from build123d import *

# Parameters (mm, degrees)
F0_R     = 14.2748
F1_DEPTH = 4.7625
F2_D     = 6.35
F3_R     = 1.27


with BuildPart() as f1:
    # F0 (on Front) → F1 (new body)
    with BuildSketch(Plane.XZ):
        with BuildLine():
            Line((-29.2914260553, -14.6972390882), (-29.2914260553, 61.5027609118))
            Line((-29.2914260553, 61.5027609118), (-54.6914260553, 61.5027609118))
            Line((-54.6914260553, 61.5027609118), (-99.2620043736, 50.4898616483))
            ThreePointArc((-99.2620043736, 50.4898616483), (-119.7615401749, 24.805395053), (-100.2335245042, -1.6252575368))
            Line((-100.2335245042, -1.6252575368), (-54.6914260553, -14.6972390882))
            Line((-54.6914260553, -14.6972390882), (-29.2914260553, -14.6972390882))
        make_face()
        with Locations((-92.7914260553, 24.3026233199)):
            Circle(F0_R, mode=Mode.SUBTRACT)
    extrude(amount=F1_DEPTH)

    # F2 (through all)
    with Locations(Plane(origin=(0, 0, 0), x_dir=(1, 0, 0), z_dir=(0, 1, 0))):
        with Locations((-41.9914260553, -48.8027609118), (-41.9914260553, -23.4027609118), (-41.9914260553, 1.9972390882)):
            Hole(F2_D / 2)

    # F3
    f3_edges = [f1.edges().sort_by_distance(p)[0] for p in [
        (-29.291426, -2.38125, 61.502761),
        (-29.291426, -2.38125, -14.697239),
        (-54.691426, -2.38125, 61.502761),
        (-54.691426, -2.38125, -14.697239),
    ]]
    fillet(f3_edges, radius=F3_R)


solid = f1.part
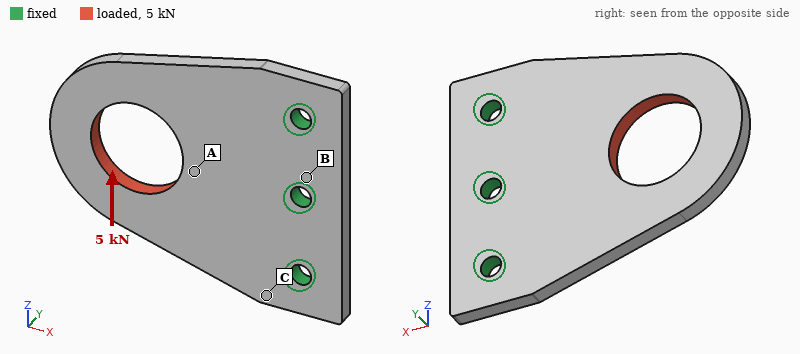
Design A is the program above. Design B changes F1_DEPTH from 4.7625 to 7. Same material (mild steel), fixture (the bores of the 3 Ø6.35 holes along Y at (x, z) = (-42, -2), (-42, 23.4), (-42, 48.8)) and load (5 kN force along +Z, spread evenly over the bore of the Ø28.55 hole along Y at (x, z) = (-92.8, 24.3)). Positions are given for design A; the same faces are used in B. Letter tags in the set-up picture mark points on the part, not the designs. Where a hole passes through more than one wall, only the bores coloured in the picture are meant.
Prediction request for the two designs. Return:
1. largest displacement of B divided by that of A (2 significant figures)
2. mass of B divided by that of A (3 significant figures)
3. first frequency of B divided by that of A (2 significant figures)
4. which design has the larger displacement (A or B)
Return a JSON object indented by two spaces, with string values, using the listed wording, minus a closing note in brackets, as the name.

{
  "largest displacement of B divided by that of A": "0.68",
  "mass of B divided by that of A": "1.47",
  "first frequency of B divided by that of A": "1.4",
  "which design has the larger displacement": "A"
}
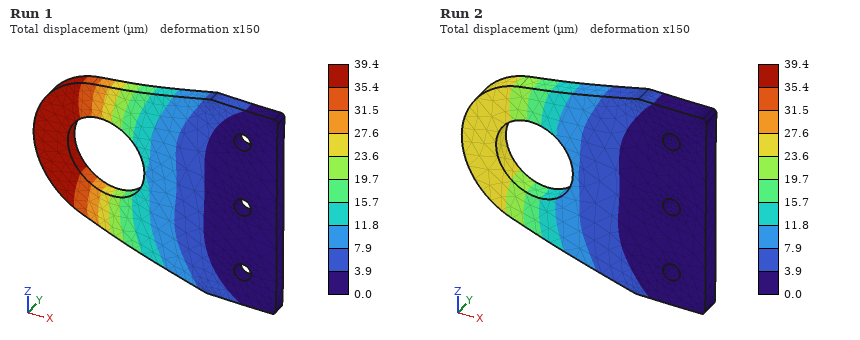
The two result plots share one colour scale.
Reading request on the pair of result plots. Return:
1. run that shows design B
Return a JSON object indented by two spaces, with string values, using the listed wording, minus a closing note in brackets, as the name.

{
  "run that shows design B": "Run 2"
}
